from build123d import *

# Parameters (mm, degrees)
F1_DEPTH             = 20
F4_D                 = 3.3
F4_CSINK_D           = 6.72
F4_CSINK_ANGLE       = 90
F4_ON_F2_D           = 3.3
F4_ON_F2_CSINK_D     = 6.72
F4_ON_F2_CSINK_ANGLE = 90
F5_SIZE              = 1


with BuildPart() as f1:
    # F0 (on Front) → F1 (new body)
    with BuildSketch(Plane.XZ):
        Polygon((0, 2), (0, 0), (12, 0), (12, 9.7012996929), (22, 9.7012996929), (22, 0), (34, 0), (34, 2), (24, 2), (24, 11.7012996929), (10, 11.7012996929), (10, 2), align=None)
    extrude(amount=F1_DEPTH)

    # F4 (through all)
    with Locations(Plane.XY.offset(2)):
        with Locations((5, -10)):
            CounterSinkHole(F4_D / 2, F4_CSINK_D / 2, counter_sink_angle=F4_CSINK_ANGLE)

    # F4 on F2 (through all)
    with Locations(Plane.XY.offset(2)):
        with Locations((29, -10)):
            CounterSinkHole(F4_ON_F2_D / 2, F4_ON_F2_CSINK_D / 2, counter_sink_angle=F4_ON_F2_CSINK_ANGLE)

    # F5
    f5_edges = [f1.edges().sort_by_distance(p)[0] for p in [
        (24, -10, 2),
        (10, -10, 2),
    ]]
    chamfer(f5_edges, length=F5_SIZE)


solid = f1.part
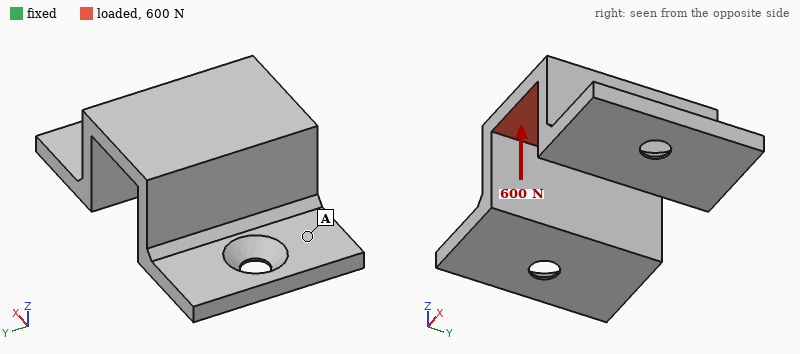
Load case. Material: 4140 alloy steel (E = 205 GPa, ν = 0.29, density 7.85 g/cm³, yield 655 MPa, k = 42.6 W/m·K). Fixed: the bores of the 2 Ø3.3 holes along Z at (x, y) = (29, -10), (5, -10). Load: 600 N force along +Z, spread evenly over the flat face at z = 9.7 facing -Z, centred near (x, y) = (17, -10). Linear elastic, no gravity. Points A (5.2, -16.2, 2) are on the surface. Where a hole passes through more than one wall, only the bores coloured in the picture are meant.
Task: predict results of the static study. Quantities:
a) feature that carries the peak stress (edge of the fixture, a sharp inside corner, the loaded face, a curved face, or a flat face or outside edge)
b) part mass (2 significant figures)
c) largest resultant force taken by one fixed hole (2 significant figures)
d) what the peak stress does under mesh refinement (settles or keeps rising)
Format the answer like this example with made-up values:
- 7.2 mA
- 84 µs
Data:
- edge of the fixture
- 16 g
- 360 N
- keeps rising
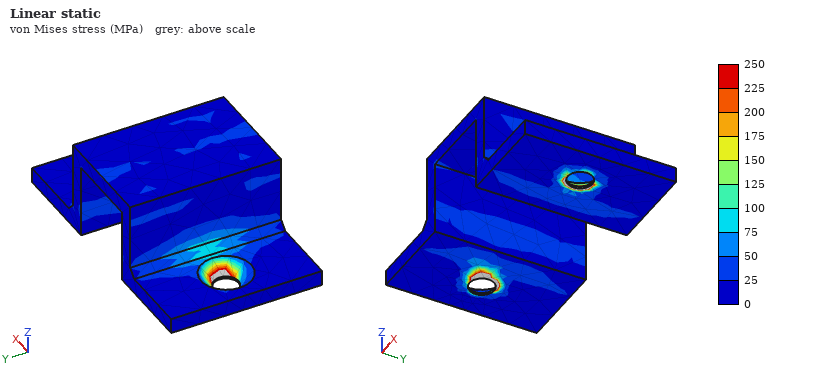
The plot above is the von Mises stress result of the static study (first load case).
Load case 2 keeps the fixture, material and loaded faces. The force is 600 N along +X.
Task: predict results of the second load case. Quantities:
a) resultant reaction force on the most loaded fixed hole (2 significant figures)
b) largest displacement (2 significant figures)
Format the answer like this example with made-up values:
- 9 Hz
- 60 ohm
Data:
- 380 N
- 17 µm
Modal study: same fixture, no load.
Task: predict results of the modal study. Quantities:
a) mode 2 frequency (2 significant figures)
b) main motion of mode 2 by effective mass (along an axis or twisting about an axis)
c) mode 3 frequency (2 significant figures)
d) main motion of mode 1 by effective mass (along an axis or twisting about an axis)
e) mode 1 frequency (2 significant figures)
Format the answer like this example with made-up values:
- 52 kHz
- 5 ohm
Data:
- 11 kHz
- along X
- 12 kHz
- along Y
- 3200 Hz
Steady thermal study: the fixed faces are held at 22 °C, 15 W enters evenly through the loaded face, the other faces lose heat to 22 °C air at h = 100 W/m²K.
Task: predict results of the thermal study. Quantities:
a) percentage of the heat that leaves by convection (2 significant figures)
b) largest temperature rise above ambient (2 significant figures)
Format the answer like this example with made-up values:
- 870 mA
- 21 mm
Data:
- 49 %
- 69 K
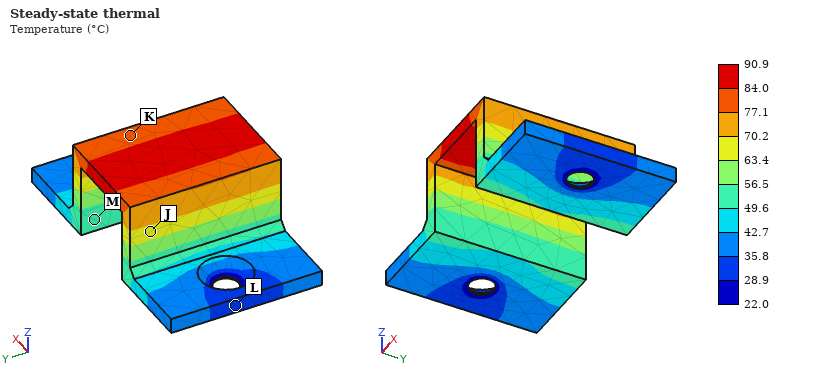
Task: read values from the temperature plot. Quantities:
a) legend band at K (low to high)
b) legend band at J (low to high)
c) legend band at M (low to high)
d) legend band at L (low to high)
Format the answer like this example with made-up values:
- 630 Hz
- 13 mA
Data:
- 77.1 to 84.0 °C
- 63.4 to 70.2 °C
- 49.6 to 56.5 °C
- 28.9 to 35.8 °C
